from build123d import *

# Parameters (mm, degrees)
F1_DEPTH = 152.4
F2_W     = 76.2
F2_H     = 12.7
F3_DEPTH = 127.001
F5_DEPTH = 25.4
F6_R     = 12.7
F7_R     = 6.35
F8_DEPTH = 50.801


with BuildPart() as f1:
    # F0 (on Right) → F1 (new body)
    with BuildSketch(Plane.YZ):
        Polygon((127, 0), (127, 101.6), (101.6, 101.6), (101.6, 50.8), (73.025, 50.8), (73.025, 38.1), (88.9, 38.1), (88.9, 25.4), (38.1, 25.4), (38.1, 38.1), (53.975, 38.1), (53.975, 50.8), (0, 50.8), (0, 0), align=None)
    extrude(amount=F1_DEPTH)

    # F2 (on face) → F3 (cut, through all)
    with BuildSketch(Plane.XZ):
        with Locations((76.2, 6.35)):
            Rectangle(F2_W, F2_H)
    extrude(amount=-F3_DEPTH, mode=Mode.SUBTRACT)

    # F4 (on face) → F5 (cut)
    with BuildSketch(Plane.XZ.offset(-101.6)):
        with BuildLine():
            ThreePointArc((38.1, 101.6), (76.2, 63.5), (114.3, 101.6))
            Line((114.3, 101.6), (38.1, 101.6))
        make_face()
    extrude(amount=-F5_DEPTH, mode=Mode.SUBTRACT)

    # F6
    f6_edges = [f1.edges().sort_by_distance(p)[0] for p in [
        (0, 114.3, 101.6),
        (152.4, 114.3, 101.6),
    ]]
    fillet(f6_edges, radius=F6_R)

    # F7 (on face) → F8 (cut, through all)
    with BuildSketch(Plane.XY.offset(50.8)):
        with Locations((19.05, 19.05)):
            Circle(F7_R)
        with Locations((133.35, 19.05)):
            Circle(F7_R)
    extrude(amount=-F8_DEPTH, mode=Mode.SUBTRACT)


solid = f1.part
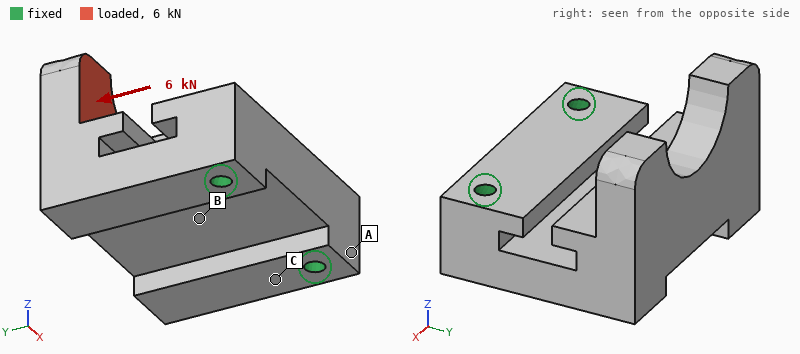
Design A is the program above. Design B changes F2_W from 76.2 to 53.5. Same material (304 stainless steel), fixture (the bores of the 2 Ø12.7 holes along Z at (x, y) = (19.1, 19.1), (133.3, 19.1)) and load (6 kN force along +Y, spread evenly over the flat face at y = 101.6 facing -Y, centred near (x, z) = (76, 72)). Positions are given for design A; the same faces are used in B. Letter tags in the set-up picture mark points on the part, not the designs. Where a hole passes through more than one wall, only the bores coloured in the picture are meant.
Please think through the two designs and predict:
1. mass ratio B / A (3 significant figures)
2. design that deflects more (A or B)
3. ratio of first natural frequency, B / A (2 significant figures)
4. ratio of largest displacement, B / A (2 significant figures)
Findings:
1.04
A
1.1
0.86
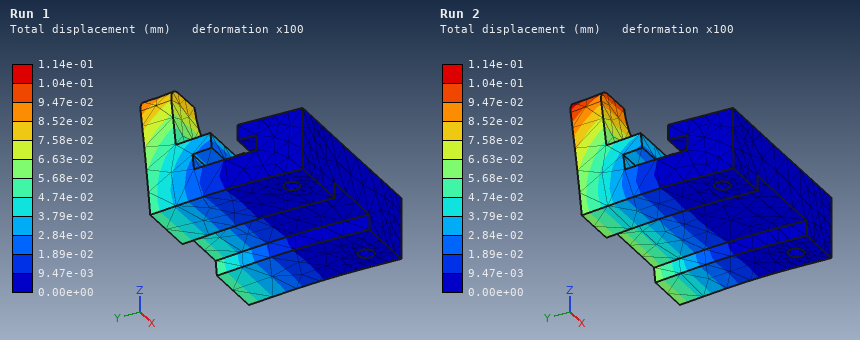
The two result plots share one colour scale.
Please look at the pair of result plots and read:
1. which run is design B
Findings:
Run 1
